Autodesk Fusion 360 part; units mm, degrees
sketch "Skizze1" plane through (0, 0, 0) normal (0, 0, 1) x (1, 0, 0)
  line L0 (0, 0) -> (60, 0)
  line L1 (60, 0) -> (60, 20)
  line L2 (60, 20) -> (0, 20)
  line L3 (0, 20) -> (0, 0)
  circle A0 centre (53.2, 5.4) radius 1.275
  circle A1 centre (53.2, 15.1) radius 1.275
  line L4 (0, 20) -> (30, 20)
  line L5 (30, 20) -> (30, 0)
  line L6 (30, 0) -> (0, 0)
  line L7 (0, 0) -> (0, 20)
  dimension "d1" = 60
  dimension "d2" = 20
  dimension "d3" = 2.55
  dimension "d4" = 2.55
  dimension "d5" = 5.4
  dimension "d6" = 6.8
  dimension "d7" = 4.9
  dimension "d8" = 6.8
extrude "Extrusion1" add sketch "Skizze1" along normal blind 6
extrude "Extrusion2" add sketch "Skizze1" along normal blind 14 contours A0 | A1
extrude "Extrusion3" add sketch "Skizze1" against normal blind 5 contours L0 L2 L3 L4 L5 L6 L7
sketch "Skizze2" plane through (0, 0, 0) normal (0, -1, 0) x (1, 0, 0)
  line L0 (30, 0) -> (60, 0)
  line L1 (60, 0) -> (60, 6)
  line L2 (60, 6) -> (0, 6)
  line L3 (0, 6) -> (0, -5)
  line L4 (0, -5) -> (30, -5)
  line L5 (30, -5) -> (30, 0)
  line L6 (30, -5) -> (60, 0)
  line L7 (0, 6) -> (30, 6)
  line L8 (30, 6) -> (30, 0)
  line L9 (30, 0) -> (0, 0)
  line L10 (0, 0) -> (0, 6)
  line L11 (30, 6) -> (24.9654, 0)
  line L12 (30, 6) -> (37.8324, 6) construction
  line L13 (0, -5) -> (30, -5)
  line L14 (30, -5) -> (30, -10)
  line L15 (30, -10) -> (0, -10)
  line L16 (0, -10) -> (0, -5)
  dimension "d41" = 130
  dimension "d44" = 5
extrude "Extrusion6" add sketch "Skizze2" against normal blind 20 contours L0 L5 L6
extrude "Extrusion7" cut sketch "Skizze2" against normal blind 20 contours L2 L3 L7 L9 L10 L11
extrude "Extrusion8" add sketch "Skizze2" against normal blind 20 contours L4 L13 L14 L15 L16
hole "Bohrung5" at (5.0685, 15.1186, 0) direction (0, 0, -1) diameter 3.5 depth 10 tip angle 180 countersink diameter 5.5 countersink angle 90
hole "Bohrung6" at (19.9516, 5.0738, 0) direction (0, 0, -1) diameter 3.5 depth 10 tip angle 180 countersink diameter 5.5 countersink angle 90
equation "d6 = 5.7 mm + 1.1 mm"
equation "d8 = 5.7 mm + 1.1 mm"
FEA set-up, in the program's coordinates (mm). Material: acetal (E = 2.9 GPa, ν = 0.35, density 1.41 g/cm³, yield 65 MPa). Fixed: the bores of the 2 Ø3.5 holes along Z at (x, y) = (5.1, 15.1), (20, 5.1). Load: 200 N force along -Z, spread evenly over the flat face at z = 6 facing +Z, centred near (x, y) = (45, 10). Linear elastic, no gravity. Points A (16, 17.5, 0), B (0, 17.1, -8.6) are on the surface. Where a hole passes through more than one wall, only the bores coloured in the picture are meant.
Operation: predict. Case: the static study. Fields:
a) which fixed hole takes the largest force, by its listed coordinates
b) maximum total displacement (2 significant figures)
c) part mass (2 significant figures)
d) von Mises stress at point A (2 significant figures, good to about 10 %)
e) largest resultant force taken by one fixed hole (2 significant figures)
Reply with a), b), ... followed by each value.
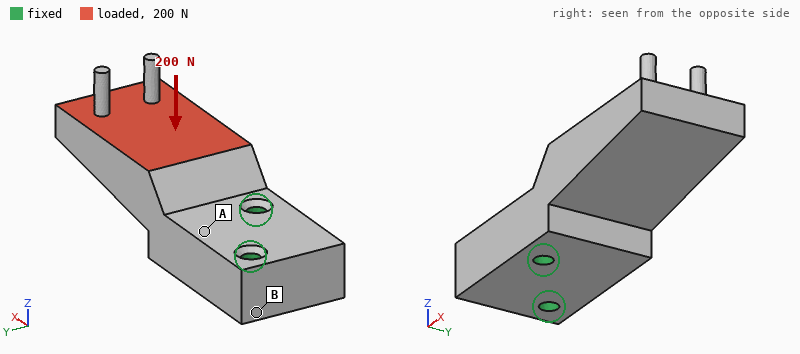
a) (20, 5.1)
b) 0.79 mm
c) 16 g
d) 6.4 MPa
e) 280 N
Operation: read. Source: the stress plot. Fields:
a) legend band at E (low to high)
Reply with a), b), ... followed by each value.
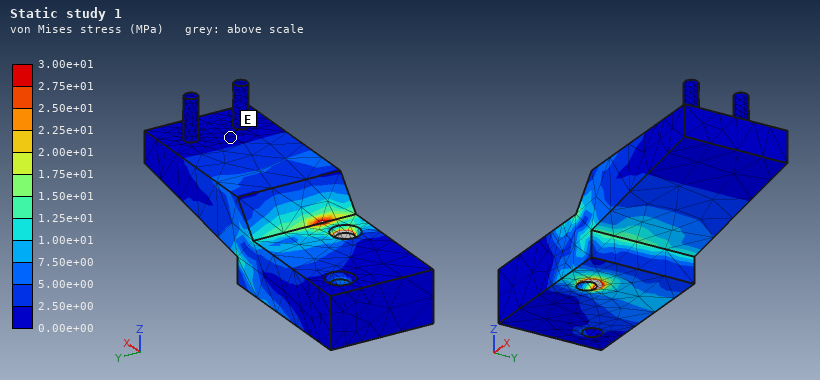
a) 0.00e+00 to 2.50e+00 MPa
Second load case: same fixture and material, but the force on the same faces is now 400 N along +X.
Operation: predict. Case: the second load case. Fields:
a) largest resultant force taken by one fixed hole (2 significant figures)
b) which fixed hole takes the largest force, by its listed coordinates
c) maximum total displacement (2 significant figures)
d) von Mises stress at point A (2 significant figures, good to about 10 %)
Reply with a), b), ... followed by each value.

a) 270 N
b) (20, 5.1)
c) 0.73 mm
d) 7.7 MPa
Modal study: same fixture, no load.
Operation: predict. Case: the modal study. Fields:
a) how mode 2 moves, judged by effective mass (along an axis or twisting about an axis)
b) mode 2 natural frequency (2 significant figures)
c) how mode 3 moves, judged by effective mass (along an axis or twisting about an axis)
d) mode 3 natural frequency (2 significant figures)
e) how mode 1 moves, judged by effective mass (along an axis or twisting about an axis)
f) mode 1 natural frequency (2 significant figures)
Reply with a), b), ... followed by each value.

a) along Y
b) 2000 Hz
c) twisting about X
d) 3700 Hz
e) along Z
f) 1200 Hz
